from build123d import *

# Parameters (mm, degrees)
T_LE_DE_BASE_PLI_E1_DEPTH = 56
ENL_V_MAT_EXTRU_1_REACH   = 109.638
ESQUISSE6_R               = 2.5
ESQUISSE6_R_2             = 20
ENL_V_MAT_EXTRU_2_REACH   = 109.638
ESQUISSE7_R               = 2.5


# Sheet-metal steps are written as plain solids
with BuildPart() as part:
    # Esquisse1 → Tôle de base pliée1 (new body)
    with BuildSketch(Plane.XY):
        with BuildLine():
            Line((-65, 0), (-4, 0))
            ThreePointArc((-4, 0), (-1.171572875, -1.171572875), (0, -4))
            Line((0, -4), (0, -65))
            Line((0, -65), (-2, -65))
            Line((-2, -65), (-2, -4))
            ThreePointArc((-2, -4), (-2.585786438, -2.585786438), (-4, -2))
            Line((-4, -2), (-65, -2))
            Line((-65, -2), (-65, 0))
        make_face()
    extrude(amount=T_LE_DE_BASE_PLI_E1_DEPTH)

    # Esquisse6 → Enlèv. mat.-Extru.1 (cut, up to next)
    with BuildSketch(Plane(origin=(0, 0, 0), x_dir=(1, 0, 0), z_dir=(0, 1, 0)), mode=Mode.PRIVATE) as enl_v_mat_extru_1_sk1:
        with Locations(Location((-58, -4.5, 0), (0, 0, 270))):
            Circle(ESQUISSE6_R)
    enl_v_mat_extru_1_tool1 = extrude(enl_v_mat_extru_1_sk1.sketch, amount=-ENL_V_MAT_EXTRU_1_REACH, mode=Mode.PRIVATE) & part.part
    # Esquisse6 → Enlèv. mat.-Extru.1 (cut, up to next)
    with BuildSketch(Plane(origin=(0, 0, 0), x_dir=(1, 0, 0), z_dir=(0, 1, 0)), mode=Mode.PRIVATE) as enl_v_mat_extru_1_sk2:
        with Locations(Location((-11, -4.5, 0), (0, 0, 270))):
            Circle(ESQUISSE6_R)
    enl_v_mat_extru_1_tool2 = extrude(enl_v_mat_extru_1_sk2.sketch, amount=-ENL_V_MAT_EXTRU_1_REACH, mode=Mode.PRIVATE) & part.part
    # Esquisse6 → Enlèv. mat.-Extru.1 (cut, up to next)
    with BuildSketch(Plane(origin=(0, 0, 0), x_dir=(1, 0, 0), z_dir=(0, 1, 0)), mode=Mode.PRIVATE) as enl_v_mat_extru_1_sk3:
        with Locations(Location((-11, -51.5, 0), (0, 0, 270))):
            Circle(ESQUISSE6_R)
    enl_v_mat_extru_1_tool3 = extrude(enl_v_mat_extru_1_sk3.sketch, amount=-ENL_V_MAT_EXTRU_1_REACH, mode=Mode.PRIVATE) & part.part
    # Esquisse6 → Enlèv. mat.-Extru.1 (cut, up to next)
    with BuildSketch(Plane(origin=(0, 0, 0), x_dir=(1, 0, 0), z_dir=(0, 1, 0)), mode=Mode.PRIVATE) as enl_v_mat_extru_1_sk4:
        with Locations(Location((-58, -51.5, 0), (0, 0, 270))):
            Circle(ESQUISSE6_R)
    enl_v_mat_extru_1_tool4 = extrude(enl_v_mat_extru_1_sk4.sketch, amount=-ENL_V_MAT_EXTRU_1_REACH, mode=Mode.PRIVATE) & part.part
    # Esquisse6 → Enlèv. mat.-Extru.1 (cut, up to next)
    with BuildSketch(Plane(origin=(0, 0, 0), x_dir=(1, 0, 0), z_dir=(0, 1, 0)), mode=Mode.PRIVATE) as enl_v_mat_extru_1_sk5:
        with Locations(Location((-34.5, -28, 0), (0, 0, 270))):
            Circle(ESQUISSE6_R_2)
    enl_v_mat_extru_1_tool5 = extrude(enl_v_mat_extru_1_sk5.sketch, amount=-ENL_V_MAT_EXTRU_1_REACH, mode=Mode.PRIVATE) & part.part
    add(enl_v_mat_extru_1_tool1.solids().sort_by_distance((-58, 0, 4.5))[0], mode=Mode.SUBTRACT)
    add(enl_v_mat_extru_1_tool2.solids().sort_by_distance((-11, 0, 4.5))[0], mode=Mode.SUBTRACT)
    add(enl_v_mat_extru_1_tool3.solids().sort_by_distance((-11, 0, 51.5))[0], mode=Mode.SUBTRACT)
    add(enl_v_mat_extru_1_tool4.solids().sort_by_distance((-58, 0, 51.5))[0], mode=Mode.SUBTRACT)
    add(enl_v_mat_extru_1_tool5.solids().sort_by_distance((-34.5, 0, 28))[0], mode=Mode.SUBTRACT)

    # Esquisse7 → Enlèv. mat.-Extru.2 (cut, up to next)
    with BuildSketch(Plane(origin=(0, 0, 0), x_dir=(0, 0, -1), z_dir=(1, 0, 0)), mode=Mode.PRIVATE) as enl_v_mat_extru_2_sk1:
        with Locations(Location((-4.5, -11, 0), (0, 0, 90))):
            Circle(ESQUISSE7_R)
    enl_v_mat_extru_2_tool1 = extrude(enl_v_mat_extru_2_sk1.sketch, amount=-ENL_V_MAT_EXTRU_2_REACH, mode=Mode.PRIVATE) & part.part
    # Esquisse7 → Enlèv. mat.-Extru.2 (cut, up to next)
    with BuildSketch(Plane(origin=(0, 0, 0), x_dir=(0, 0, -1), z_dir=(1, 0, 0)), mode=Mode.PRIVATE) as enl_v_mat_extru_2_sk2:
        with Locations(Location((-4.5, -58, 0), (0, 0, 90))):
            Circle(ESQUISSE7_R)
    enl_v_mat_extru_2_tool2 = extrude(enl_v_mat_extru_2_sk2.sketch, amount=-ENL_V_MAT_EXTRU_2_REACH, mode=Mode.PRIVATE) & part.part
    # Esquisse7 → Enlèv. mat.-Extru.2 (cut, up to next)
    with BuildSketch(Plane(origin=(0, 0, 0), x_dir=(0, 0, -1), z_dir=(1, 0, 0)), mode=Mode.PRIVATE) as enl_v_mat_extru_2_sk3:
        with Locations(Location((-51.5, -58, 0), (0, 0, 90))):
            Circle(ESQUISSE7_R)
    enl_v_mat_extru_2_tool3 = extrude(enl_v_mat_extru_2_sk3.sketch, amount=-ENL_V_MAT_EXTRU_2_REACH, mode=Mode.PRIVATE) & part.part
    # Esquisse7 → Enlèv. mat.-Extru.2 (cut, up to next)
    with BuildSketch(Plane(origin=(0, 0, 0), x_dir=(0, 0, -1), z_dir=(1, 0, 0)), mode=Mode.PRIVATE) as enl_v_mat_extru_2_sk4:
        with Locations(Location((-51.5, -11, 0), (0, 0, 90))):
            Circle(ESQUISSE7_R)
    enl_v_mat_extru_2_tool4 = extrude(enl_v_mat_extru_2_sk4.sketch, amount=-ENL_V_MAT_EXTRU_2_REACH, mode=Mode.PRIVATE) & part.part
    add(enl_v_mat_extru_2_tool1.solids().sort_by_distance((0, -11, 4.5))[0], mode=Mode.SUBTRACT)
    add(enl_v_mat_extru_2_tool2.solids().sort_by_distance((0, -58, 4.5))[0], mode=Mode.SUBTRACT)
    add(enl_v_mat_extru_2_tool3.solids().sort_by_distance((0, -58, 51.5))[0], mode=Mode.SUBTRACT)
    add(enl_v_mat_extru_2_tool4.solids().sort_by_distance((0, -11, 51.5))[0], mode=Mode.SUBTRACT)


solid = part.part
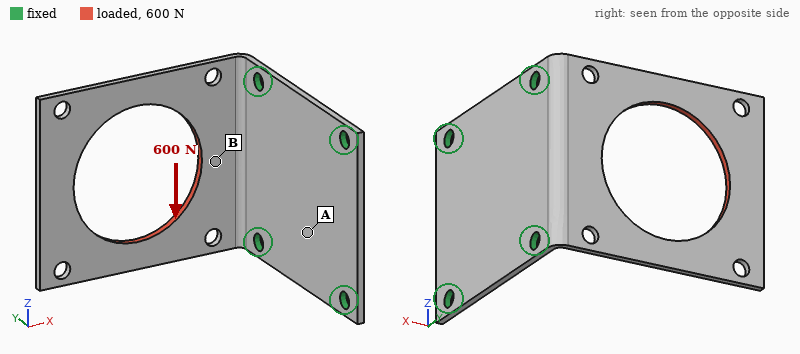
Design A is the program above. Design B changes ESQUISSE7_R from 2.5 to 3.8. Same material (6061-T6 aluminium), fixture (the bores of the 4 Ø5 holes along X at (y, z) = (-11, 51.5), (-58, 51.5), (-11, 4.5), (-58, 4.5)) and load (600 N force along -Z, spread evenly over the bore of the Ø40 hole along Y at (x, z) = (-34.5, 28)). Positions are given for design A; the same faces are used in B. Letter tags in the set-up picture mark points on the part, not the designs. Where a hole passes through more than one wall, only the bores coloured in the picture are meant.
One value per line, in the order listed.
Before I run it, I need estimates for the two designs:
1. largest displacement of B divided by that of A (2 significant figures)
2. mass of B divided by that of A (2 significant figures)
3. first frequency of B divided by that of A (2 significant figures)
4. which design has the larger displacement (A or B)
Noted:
0.73
0.98
1.0
A
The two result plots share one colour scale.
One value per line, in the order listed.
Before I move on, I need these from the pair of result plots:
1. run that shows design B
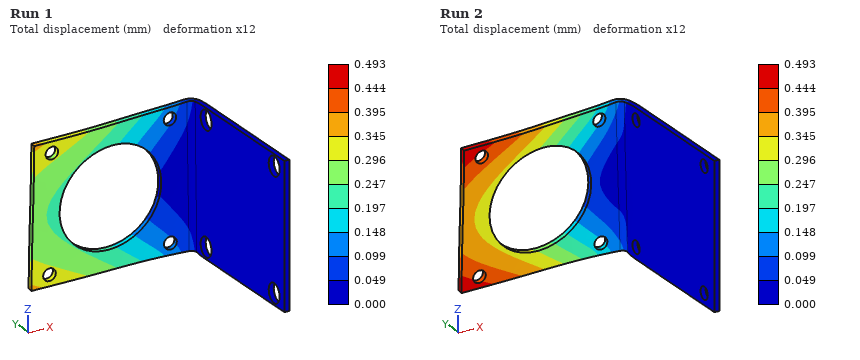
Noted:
Run 1
